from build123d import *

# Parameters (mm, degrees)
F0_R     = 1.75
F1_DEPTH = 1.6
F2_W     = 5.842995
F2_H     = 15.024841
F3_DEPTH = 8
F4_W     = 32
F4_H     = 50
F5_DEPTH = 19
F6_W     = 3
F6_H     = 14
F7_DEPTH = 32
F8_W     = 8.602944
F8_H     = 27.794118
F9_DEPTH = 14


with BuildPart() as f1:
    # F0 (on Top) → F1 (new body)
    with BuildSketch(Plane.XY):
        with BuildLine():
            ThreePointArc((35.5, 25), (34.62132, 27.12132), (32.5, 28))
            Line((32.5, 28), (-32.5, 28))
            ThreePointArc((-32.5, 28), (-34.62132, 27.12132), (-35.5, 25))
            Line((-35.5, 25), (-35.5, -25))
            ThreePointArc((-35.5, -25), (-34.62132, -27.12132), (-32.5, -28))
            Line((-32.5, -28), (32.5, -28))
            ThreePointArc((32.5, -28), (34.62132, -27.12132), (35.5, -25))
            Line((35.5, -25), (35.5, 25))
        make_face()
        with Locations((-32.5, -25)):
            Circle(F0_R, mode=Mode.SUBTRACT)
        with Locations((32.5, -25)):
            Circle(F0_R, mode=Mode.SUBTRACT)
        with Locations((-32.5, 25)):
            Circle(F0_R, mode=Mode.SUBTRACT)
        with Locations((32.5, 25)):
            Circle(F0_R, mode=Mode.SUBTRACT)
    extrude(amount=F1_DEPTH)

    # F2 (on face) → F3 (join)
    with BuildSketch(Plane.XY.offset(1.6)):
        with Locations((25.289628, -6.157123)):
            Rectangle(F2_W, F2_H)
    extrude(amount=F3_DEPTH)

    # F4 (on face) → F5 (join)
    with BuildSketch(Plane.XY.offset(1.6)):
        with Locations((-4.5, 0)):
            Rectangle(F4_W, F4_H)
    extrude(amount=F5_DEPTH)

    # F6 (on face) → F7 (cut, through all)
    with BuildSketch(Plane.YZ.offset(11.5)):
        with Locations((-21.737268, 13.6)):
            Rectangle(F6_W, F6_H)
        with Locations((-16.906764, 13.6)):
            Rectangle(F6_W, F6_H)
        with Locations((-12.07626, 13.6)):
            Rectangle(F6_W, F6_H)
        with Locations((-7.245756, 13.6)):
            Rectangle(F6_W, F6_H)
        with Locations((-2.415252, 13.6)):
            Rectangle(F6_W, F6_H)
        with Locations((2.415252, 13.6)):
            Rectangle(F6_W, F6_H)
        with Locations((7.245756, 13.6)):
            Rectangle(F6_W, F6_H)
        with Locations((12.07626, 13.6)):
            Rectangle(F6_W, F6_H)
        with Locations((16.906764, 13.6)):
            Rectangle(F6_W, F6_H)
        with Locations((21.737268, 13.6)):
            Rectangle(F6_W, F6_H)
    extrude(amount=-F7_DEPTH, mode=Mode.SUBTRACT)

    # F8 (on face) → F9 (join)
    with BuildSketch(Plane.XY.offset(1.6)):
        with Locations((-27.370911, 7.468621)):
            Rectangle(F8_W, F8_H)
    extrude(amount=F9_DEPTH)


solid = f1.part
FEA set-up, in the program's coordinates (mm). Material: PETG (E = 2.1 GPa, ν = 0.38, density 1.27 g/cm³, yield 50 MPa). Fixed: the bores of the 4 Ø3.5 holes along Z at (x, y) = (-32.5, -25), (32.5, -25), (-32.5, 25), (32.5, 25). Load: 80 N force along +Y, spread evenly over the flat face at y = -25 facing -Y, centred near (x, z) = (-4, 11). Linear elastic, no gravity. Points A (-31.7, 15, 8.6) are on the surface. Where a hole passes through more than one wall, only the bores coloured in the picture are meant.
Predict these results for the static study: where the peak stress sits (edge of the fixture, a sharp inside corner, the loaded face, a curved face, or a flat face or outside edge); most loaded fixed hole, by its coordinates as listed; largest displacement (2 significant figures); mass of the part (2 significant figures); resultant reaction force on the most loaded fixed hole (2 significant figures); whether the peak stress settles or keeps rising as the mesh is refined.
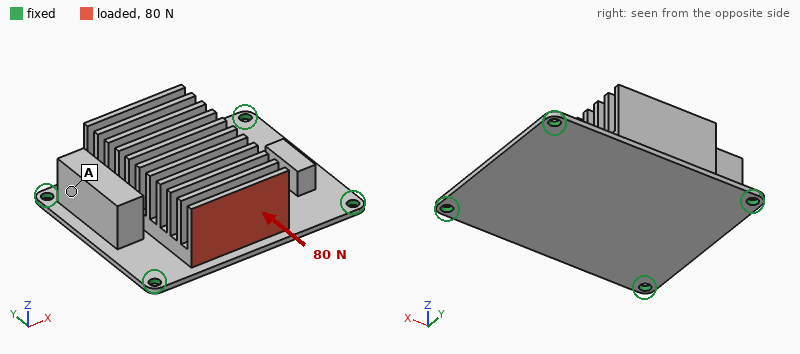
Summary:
edge of the fixture
(-32.5, 25)
0.97 mm
35 g
44 N
keeps rising
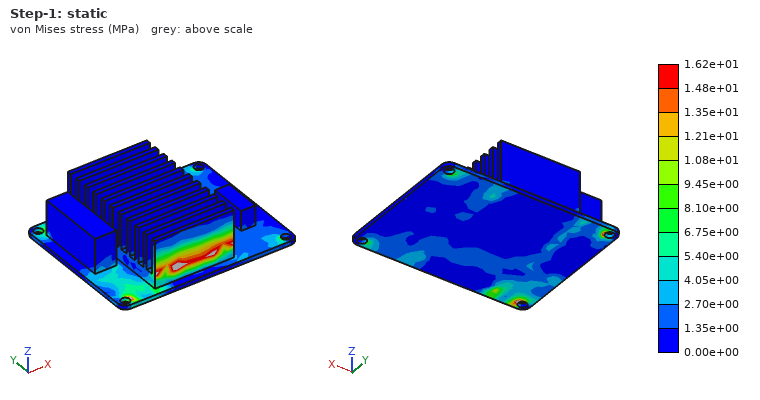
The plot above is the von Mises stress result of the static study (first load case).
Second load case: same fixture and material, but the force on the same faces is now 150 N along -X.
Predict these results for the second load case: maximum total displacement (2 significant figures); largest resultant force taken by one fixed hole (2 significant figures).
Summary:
0.91 mm
55 N
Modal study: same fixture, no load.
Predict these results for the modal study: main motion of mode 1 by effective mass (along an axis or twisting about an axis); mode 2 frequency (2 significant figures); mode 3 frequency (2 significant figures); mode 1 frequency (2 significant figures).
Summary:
along Z
520 Hz
730 Hz
310 Hz
